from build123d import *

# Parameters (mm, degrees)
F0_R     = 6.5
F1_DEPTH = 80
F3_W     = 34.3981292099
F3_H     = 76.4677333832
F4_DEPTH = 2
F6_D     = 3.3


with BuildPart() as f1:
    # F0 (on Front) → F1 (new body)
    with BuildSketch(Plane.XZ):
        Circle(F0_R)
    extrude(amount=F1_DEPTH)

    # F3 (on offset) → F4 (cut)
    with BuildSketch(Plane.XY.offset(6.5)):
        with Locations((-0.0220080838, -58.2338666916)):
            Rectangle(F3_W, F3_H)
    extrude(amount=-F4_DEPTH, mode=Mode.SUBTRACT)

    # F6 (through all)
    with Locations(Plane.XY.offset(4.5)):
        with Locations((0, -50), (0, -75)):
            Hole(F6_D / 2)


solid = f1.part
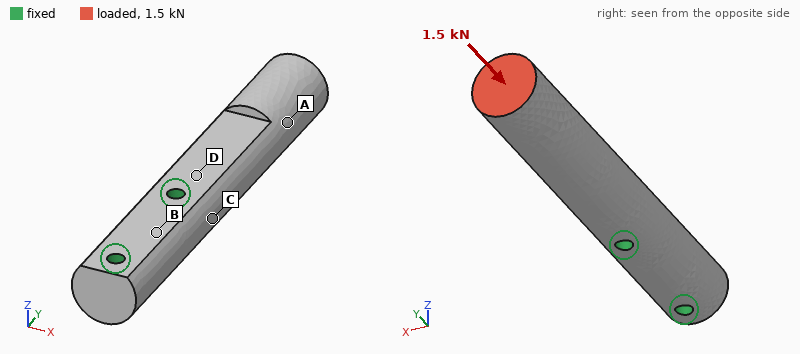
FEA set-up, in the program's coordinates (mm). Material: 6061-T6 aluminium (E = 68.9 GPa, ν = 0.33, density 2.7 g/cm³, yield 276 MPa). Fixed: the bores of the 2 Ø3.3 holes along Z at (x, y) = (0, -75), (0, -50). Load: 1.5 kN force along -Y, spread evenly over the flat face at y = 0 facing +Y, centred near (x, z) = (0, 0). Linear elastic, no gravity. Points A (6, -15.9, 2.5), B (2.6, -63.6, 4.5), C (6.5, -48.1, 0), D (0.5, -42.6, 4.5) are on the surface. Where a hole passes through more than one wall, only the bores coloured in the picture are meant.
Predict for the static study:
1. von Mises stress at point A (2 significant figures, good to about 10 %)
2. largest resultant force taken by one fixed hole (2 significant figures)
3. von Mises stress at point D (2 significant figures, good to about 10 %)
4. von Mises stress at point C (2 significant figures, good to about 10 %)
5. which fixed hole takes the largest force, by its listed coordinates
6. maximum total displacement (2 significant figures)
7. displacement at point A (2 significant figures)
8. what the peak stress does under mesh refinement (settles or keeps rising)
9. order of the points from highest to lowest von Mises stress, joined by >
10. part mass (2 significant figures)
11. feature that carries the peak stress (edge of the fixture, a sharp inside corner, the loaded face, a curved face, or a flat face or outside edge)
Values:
13 MPa
1.4 kN
19 MPa
6.7 MPa
(0, -50)
19 µm
11 µm
keeps rising
D > A > C > B
26 g
edge of the fixture
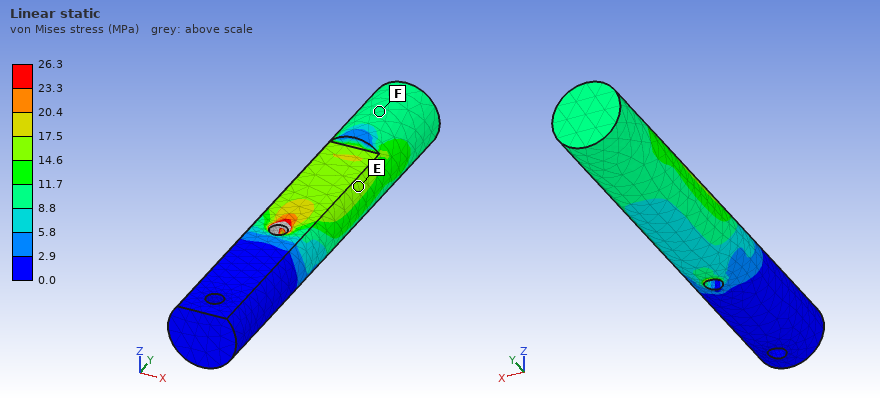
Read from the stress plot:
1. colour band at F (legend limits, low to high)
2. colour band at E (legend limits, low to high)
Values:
8.8 to 11.7 MPa
14.6 to 17.5 MPa
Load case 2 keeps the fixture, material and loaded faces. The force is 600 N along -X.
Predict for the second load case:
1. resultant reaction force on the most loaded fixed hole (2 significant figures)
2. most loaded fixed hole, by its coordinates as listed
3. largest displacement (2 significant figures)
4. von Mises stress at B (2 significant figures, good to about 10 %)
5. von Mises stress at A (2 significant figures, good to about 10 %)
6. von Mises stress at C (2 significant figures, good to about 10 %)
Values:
1.3 kN
(0, -50)
0.35 mm
17 MPa
41 MPa
120 MPa
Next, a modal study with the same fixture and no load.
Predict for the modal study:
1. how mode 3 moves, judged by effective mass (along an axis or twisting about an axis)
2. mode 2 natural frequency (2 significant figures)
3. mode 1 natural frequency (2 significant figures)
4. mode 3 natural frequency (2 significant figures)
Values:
twisting about Y
3100 Hz
3000 Hz
14 kHz
